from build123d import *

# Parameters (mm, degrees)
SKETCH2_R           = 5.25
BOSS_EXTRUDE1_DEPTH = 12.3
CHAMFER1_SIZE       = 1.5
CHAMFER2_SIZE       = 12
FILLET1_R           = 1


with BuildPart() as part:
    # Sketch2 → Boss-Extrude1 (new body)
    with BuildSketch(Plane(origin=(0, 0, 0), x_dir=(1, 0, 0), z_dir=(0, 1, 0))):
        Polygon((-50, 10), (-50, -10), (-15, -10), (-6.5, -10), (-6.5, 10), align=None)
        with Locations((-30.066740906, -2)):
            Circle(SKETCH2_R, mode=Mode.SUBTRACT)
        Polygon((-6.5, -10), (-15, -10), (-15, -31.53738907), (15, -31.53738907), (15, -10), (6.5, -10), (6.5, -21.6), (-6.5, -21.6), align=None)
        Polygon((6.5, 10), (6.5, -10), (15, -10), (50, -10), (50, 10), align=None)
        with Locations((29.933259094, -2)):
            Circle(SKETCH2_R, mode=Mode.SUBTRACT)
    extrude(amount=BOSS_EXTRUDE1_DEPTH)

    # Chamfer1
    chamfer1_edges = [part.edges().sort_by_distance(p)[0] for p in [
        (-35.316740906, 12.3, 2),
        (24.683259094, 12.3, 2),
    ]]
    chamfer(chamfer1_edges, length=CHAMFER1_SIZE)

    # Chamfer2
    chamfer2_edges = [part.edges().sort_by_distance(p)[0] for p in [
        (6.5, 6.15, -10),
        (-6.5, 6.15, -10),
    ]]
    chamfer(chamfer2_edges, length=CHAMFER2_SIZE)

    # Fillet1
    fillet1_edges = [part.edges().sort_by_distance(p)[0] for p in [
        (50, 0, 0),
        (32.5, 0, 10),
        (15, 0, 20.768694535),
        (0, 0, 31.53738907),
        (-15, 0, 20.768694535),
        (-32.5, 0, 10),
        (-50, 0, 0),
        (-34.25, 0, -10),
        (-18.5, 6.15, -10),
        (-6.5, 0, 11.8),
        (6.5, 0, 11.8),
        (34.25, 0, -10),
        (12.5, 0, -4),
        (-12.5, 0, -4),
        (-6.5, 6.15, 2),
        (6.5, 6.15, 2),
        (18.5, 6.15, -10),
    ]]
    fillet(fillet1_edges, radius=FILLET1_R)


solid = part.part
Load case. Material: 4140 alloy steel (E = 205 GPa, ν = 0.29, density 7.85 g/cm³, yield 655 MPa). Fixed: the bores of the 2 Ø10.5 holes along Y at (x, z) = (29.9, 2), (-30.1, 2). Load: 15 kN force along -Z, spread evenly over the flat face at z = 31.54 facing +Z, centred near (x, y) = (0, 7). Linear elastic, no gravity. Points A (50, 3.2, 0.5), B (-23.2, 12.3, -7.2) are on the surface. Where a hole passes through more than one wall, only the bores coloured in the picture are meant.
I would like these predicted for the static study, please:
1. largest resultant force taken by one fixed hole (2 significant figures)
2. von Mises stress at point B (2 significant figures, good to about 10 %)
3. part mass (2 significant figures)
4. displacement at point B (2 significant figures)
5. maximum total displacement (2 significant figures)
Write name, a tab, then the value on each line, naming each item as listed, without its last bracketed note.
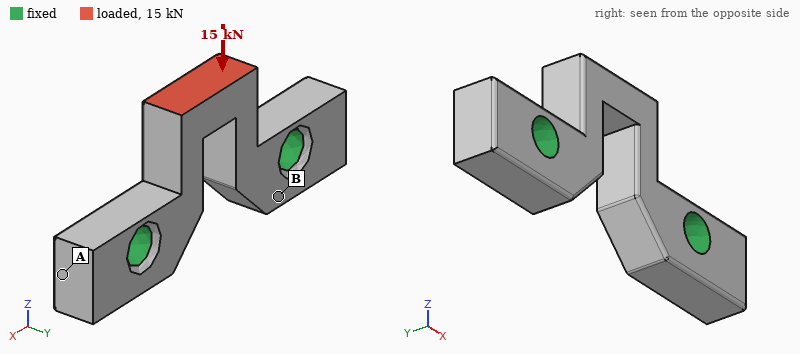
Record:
largest resultant force taken by one fixed hole	7.8 kN
von Mises stress at point B	52 MPa
part mass	180 g
displacement at point B	5.0 µm
maximum total displacement	27 µm
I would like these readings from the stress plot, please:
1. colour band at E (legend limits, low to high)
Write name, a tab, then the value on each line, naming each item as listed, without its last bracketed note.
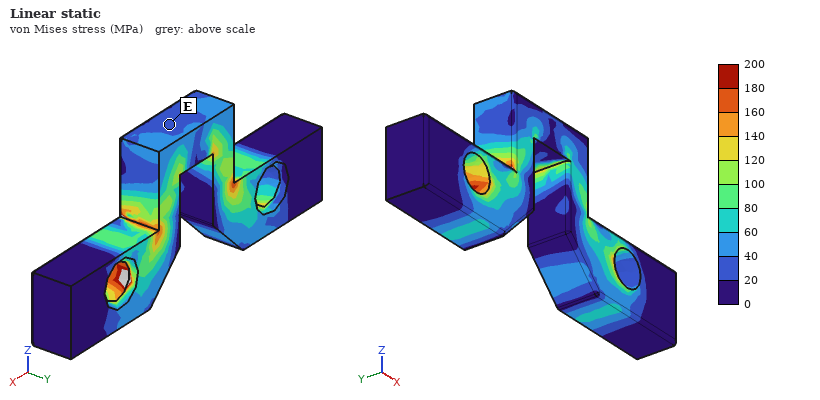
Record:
colour band at E	20 to 40 MPa
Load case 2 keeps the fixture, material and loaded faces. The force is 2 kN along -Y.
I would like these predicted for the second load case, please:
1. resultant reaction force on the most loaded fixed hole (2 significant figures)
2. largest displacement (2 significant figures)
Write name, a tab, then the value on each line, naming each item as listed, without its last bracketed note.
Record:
resultant reaction force on the most loaded fixed hole	1.0 kN
largest displacement	57 µm
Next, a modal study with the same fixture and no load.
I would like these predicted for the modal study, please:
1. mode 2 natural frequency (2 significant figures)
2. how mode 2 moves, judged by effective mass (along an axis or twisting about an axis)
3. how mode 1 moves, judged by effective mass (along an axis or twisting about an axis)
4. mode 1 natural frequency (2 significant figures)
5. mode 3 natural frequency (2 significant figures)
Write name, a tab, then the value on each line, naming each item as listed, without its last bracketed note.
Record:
mode 2 natural frequency	13 kHz
how mode 2 moves, judged by effective mass	along X
how mode 1 moves, judged by effective mass	along Y
mode 1 natural frequency	6300 Hz
mode 3 natural frequency	14 kHz
